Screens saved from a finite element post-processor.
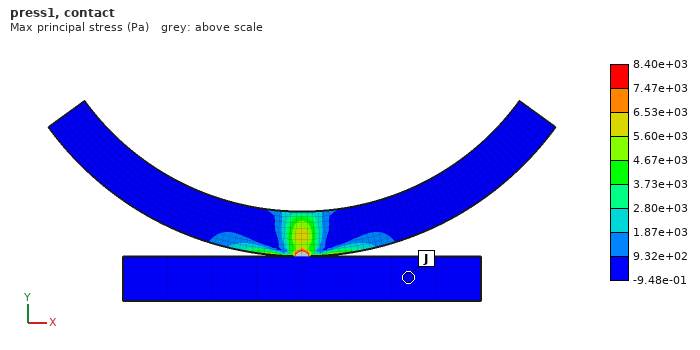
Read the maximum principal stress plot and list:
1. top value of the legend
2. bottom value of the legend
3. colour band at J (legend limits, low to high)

8.40e+03 Pa
-9.48e-01 Pa
-9.48e-01 to 9.32e+02 Pa
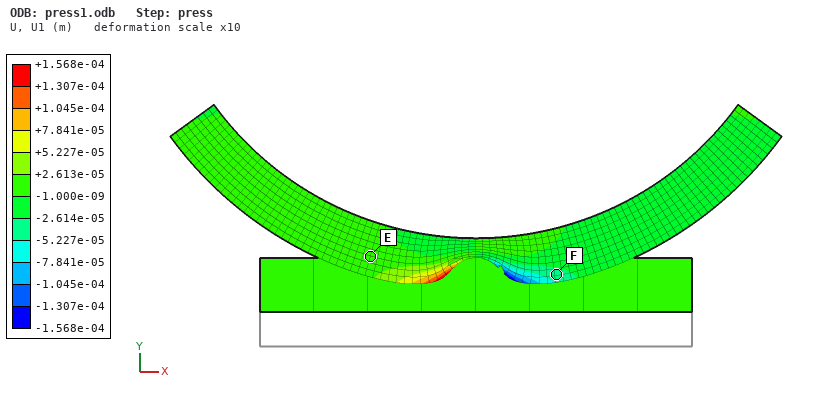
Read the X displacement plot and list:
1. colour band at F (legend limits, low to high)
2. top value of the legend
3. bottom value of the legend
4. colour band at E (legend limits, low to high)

-5.227e-05 to -2.614e-05 m
+1.568e-04 m
-1.568e-04 m
-1.000e-09 to +2.613e-05 m
